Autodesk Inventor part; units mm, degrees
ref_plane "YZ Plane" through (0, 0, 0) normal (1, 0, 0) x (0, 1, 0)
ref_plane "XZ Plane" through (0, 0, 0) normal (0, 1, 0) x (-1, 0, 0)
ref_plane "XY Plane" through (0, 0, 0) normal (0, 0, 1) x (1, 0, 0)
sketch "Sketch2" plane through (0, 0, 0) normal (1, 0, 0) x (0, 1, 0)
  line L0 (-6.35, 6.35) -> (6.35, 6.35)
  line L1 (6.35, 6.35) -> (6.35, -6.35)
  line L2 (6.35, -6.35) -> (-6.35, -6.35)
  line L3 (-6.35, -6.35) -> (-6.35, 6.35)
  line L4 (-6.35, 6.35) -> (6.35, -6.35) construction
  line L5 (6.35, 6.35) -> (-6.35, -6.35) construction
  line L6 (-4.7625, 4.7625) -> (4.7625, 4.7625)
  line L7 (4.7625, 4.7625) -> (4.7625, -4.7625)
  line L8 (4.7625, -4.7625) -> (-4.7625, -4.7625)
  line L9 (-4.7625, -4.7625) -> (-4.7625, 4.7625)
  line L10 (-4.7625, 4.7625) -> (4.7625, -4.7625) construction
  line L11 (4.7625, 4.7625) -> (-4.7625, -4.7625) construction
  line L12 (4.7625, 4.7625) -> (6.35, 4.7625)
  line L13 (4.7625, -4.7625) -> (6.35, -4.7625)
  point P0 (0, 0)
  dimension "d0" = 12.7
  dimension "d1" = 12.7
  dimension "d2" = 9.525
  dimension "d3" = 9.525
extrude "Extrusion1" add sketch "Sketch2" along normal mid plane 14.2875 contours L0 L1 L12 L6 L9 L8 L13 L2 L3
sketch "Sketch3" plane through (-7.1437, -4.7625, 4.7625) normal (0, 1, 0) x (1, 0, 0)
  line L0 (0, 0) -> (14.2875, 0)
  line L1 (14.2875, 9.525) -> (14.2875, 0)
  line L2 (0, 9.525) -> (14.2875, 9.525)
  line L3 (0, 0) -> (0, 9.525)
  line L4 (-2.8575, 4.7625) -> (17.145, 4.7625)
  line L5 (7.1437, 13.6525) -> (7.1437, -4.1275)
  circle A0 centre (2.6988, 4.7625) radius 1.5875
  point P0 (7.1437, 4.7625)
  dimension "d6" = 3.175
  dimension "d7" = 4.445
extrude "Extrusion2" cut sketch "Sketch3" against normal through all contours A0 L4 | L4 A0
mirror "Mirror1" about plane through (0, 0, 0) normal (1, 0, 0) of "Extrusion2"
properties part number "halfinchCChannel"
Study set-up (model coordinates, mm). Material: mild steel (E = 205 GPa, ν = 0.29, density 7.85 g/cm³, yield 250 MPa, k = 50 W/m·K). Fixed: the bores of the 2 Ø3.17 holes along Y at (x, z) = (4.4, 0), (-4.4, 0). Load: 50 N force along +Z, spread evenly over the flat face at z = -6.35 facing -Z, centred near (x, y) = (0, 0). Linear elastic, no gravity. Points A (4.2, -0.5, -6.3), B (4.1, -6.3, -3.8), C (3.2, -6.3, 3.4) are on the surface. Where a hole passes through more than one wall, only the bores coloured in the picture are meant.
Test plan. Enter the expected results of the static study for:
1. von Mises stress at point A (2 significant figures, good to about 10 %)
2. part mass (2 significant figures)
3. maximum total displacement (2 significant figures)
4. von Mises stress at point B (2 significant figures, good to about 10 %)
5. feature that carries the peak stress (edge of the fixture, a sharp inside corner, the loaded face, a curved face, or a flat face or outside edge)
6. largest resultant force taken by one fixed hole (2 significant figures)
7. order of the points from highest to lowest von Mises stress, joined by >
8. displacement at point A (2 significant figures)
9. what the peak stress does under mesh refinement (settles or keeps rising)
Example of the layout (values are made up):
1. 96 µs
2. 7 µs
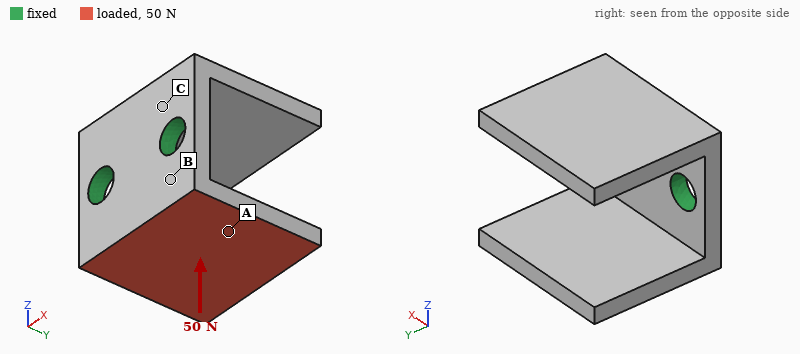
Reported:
1. 15 MPa
2. 6.0 g
3. 23 µm
4. 40 MPa
5. edge of the fixture
6. 26 N
7. B > A > C
8. 9.1 µm
9. keeps rising
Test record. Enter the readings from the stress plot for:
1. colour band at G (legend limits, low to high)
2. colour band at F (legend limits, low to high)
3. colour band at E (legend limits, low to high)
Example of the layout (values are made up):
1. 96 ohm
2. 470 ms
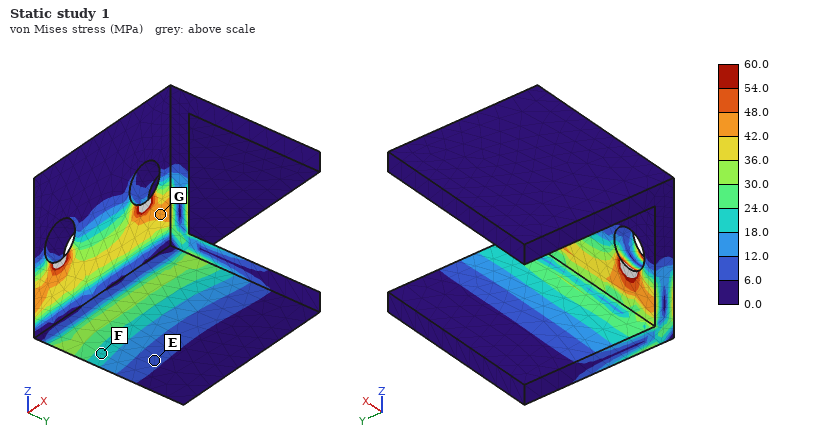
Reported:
1. 42.0 to 48.0 MPa
2. 18.0 to 24.0 MPa
3. 6.0 to 12.0 MPa
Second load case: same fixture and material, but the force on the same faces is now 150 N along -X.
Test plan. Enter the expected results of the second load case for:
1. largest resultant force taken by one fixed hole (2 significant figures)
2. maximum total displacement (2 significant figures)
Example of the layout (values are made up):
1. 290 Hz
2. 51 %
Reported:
1. 140 N
2. 9.4 µm
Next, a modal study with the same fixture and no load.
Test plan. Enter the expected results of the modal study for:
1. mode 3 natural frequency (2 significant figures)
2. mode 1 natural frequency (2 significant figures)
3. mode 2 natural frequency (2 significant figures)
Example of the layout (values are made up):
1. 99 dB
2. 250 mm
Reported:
1. 13 kHz
2. 6000 Hz
3. 6000 Hz
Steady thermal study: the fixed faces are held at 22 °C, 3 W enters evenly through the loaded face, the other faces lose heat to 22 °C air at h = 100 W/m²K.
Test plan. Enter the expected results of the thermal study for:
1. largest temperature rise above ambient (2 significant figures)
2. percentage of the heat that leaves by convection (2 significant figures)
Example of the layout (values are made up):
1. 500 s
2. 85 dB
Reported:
1. 22 K
2. 16 %
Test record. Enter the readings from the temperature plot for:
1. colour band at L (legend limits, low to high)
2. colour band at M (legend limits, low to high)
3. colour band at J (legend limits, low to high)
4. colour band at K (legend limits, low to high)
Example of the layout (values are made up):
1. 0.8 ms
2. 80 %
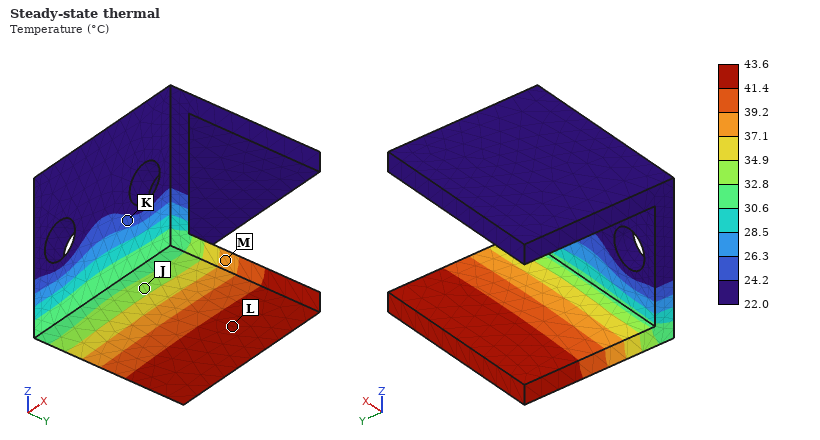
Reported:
1. 41.4 to 43.6 °C
2. 37.1 to 39.2 °C
3. 32.8 to 34.9 °C
4. 24.2 to 26.3 °C
